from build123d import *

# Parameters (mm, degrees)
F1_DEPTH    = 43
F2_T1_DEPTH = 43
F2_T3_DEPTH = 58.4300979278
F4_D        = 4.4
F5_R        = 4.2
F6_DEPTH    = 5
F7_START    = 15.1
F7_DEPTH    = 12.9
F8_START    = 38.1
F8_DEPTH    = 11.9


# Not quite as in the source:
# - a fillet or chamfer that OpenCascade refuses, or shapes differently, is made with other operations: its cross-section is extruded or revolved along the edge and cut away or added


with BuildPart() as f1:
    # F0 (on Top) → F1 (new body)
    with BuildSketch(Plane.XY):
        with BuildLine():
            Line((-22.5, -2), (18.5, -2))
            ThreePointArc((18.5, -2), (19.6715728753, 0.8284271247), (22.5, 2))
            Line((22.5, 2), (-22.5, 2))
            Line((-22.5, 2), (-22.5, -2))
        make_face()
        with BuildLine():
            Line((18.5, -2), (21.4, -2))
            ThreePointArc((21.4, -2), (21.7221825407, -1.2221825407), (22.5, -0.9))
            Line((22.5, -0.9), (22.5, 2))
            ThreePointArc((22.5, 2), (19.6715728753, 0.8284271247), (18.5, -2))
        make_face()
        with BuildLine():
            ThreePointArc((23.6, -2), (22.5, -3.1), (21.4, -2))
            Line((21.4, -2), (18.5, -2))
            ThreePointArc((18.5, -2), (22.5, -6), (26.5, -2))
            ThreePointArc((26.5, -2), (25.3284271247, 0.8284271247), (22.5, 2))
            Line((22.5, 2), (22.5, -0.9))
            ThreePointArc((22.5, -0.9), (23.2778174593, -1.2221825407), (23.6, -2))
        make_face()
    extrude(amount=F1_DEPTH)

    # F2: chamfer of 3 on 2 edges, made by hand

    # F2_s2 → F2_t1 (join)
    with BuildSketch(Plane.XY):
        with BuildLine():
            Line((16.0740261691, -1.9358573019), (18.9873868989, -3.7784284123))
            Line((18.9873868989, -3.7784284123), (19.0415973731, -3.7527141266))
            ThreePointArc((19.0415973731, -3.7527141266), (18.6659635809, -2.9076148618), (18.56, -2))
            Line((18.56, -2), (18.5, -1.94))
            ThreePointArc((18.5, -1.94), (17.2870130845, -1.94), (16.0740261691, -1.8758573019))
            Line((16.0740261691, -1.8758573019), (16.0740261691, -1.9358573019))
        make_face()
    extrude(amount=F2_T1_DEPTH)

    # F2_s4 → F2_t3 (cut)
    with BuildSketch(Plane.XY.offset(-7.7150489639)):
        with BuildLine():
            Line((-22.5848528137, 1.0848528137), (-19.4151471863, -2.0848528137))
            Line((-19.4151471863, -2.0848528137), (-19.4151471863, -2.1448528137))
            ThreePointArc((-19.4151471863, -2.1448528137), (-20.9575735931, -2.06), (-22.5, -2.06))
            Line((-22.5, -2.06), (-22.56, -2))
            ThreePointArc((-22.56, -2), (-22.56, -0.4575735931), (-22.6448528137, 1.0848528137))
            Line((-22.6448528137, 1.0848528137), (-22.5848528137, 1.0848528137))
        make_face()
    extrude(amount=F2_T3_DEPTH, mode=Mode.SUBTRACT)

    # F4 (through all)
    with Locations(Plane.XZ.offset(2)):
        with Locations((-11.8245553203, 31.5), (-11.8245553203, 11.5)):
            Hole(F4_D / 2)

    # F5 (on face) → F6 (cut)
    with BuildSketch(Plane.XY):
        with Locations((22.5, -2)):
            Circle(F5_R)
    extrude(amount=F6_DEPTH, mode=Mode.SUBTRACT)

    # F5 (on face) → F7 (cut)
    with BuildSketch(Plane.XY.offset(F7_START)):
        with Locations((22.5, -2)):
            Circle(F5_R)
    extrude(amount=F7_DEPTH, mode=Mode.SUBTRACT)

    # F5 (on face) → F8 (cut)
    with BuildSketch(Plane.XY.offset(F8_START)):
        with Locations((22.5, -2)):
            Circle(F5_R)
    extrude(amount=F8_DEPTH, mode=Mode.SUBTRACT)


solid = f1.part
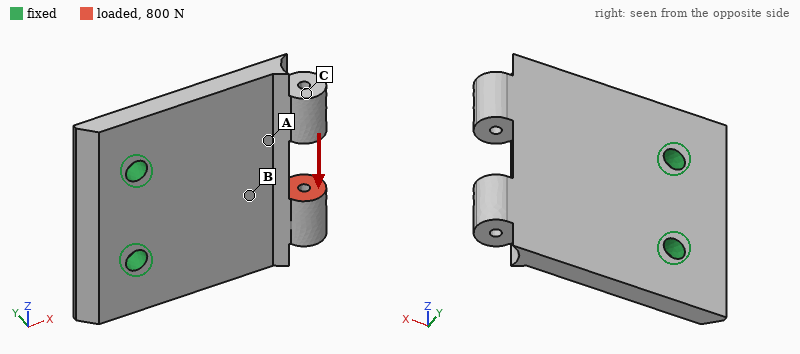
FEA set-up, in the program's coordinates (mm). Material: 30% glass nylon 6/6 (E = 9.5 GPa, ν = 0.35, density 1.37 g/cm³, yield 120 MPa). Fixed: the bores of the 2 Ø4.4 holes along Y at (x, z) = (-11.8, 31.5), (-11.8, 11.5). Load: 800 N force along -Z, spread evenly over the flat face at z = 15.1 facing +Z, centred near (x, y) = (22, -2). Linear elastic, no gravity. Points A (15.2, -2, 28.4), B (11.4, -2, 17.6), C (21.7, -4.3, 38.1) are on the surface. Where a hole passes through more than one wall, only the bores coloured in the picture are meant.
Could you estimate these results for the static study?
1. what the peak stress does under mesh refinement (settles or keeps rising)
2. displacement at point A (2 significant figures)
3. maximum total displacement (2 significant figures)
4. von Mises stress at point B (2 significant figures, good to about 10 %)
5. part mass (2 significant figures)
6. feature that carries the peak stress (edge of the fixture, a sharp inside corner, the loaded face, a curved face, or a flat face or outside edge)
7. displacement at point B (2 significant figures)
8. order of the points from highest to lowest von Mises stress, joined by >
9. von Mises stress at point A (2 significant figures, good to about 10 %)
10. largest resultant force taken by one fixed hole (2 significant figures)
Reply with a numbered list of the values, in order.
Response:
1. keeps rising
2. 0.14 mm
3. 0.37 mm
4. 32 MPa
5. 11 g
6. a sharp inside corner
7. 0.11 mm
8. B > A > C
9. 16 MPa
10. 1.3 kN
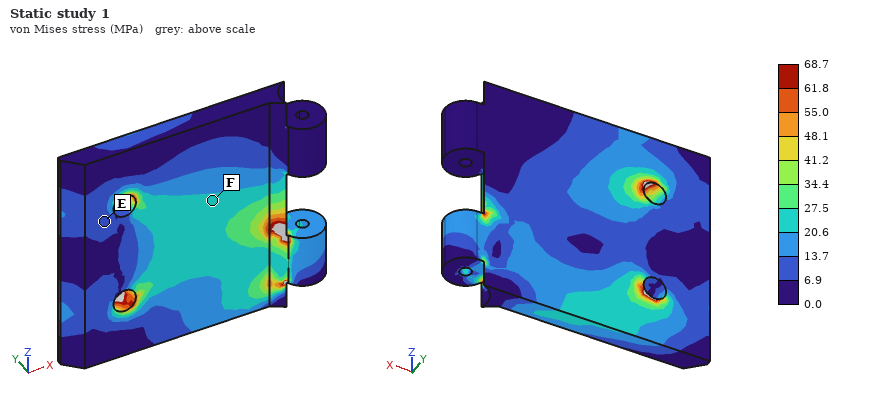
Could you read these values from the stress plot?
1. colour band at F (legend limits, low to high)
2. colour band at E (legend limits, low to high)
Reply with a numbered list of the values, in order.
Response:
1. 20.6 to 27.5 MPa
2. 6.9 to 13.7 MPa
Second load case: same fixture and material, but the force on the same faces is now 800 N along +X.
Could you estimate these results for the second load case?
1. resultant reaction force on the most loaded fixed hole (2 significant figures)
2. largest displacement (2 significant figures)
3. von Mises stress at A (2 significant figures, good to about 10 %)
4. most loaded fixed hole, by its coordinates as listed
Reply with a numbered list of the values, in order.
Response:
1. 630 N
2. 0.67 mm
3. 9.0 MPa
4. (-11.8, 11.5)
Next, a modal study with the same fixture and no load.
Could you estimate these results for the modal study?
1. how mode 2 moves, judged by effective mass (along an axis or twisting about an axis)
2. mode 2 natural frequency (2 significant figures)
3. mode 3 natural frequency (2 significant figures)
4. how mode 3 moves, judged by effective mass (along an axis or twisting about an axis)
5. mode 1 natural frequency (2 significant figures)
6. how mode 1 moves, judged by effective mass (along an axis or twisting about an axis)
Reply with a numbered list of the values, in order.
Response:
1. twisting about X
2. 2400 Hz
3. 6100 Hz
4. along Z
5. 1300 Hz
6. along Y
